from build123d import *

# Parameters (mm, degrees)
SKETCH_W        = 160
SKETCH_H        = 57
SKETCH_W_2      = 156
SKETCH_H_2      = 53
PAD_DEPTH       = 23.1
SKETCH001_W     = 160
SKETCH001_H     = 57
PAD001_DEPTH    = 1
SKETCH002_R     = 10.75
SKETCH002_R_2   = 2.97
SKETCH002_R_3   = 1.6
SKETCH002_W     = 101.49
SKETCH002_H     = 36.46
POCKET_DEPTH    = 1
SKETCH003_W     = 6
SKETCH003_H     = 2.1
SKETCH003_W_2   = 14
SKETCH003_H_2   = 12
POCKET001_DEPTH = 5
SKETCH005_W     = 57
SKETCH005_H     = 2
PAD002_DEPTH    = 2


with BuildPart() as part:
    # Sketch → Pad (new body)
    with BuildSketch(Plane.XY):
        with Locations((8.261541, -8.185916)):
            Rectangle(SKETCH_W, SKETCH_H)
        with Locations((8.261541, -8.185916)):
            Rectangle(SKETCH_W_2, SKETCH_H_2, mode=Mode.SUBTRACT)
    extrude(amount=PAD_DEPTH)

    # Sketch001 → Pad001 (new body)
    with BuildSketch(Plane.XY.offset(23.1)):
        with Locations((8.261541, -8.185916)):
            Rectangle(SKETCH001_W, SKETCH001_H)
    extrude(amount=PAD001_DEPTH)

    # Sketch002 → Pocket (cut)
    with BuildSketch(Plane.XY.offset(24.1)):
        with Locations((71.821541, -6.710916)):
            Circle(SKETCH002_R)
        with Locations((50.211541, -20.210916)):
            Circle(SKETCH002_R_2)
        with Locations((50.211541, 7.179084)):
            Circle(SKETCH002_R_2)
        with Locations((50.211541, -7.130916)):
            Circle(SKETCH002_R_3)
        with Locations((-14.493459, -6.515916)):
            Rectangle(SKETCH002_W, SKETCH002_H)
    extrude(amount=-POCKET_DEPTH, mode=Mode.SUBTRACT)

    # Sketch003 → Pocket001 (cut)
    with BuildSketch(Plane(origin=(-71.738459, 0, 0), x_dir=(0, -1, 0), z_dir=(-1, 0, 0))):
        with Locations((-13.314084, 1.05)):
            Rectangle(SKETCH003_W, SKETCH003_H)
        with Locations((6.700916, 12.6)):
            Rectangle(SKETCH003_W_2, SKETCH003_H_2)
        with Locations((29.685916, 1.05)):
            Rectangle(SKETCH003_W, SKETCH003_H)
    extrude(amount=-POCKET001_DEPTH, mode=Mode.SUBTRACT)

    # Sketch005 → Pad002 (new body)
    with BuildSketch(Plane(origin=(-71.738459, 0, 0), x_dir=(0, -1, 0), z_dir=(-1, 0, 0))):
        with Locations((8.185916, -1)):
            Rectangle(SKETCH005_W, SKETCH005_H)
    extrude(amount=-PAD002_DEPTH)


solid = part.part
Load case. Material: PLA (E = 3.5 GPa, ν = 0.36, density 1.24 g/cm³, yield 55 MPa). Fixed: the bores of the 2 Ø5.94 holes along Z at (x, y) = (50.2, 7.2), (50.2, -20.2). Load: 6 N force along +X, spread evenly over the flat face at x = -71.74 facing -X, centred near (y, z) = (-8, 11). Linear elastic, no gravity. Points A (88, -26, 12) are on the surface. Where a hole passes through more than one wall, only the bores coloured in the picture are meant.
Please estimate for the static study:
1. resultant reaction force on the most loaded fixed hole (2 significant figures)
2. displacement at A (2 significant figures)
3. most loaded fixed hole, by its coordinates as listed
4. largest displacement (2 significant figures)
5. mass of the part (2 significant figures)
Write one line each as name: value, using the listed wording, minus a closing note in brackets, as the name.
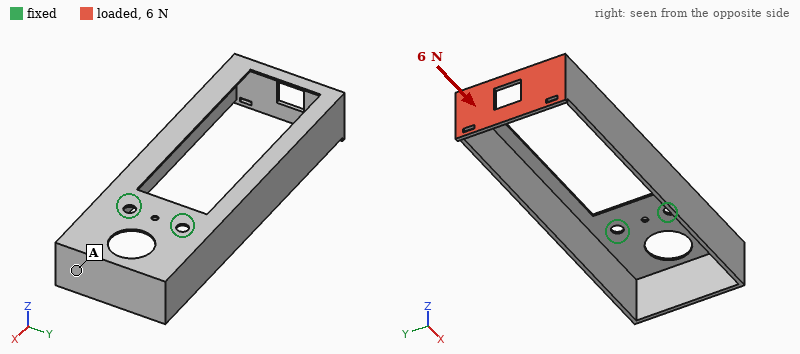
resultant reaction force on the most loaded fixed hole: 3.4 N
displacement at A: 0.54 mm
most loaded fixed hole, by its coordinates as listed: (50.2, -20.2)
largest displacement: 1.7 mm
mass of the part: 30 g
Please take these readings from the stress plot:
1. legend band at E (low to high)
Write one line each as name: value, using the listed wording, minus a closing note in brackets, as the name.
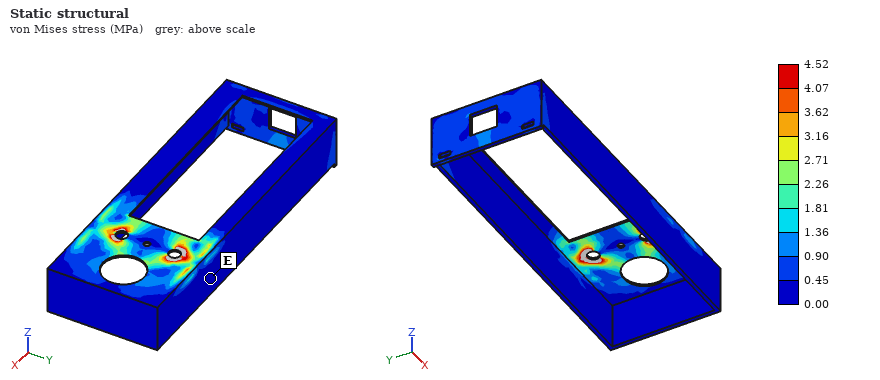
legend band at E: 0.00 to 0.45 MPa
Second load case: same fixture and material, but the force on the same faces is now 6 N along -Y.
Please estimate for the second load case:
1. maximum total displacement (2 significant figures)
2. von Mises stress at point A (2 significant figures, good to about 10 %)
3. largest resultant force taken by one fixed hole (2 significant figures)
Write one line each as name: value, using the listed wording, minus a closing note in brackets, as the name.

maximum total displacement: 1.8 mm
von Mises stress at point A: 0.73 MPa
largest resultant force taken by one fixed hole: 21 N
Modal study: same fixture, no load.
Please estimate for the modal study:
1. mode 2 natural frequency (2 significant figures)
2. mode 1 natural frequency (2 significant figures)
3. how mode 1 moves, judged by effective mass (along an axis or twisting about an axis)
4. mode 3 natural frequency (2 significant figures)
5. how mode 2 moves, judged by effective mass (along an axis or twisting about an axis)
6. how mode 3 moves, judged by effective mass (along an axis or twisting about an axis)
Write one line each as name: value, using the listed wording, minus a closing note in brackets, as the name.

mode 2 natural frequency: 93 Hz
mode 1 natural frequency: 31 Hz
how mode 1 moves, judged by effective mass: along Z
mode 3 natural frequency: 160 Hz
how mode 2 moves, judged by effective mass: along Y
how mode 3 moves, judged by effective mass: along Y
